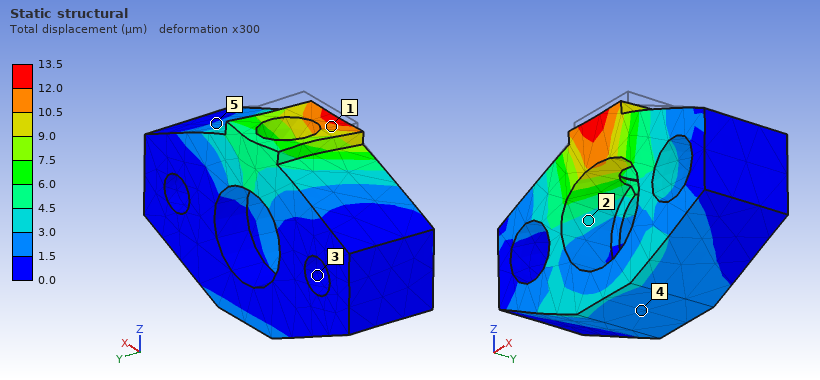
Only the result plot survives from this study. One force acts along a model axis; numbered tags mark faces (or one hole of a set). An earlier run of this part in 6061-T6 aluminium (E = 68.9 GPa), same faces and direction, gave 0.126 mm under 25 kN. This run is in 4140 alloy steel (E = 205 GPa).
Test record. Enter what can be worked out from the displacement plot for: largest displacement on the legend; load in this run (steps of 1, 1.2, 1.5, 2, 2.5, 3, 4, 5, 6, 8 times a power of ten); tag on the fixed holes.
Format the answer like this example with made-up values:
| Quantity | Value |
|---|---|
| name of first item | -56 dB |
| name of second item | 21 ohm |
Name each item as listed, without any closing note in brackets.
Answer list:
| Quantity | Value |
|---|---|
| largest displacement on the legend | 13.5 µm |
| load in this run | 8 kN |
| tag on the fixed holes | 3 |
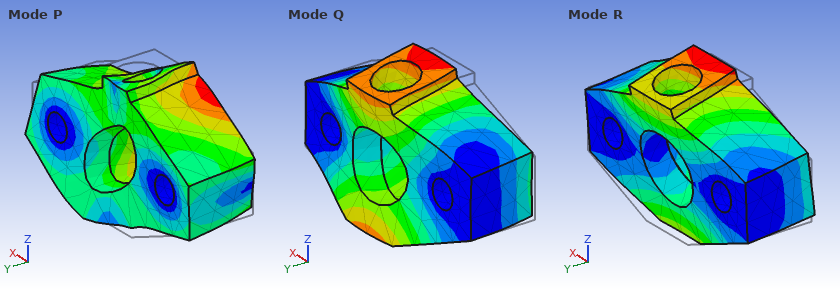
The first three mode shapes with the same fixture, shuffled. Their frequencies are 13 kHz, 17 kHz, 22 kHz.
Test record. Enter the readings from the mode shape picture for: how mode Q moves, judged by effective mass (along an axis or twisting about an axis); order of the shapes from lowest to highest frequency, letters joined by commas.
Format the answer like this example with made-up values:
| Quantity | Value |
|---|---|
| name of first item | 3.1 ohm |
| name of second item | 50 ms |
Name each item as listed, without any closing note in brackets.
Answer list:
| Quantity | Value |
|---|---|
| how mode Q moves, judged by effective mass | along Y |
| order of the shapes from lowest to highest frequency, letters joined by commas | R, Q, P |
